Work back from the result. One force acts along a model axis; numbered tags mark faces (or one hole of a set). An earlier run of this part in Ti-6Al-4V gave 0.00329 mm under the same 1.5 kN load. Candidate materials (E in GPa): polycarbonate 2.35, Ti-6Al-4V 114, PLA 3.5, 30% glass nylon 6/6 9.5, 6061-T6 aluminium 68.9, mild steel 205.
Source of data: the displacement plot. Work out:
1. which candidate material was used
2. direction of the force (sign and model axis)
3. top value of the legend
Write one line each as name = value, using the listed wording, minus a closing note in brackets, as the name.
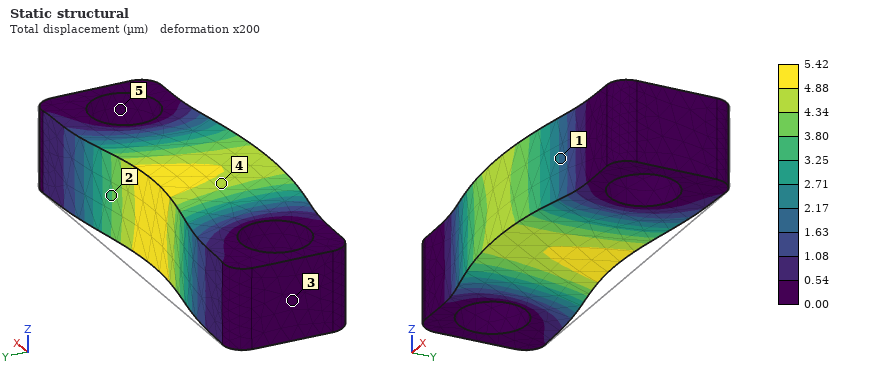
which candidate material was used = 6061-T6 aluminium
direction of the force = -Y
top value of the legend = 5.42 µm
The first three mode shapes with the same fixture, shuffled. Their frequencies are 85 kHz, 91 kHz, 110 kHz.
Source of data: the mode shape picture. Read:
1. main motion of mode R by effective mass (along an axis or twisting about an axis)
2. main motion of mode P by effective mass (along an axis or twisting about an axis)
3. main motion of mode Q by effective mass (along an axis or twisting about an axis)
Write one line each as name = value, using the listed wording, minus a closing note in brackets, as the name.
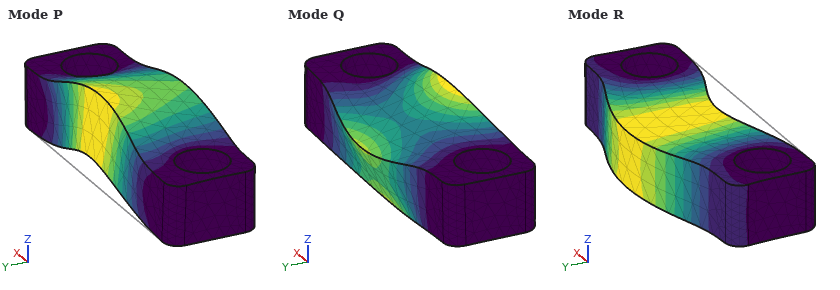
main motion of mode R by effective mass = along Y
main motion of mode P by effective mass = along Z
main motion of mode Q by effective mass = twisting about X
